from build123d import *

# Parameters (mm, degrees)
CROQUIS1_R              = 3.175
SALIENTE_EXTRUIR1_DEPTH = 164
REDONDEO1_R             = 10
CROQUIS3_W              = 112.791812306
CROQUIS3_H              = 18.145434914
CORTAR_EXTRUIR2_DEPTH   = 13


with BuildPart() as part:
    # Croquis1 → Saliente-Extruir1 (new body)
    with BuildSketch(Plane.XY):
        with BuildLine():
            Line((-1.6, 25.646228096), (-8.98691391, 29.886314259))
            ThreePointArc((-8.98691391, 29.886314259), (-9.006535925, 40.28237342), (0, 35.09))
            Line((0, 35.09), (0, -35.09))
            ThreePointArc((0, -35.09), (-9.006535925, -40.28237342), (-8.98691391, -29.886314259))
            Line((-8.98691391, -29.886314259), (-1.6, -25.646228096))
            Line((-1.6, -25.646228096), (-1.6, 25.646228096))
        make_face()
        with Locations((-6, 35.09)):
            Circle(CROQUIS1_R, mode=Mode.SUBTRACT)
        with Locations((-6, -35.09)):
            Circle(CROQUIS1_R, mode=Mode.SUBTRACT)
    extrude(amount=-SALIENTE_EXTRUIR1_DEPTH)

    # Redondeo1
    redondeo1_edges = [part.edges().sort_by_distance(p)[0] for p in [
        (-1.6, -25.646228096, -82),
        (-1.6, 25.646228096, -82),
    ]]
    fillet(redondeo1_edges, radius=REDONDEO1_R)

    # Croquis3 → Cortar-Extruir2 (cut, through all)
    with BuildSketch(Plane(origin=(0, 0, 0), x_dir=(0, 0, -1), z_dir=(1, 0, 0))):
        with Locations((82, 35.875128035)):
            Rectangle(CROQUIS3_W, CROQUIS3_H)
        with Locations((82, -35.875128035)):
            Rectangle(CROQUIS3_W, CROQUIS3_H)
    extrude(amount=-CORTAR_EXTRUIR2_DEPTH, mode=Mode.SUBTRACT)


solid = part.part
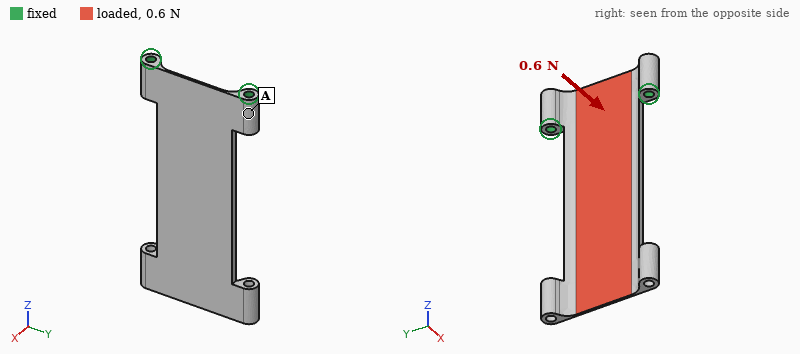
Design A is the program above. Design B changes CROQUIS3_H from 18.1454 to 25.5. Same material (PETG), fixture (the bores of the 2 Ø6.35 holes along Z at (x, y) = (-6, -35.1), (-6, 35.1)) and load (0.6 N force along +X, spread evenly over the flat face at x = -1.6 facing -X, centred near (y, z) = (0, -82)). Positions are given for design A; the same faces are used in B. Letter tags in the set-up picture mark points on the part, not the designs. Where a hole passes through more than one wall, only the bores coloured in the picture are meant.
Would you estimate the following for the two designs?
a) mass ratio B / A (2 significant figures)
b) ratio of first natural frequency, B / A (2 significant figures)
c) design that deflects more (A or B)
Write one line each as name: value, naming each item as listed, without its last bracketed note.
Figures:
mass ratio B / A: 0.90
ratio of first natural frequency, B / A: 0.56
design that deflects more: B
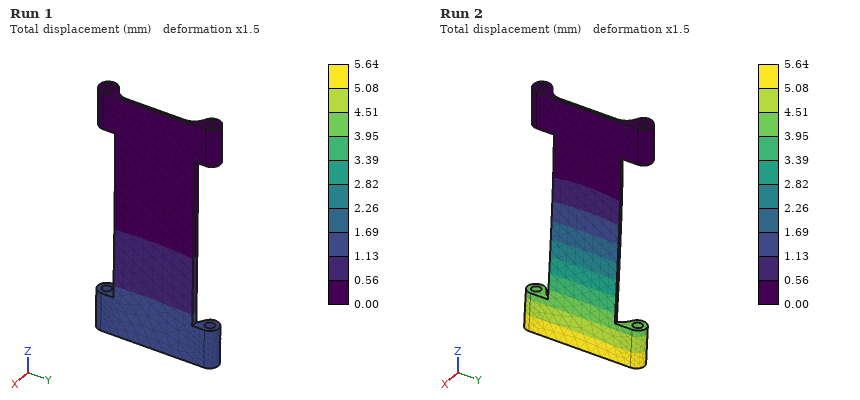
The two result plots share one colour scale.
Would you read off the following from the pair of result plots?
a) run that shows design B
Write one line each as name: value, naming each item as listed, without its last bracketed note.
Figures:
run that shows design B: Run 2
